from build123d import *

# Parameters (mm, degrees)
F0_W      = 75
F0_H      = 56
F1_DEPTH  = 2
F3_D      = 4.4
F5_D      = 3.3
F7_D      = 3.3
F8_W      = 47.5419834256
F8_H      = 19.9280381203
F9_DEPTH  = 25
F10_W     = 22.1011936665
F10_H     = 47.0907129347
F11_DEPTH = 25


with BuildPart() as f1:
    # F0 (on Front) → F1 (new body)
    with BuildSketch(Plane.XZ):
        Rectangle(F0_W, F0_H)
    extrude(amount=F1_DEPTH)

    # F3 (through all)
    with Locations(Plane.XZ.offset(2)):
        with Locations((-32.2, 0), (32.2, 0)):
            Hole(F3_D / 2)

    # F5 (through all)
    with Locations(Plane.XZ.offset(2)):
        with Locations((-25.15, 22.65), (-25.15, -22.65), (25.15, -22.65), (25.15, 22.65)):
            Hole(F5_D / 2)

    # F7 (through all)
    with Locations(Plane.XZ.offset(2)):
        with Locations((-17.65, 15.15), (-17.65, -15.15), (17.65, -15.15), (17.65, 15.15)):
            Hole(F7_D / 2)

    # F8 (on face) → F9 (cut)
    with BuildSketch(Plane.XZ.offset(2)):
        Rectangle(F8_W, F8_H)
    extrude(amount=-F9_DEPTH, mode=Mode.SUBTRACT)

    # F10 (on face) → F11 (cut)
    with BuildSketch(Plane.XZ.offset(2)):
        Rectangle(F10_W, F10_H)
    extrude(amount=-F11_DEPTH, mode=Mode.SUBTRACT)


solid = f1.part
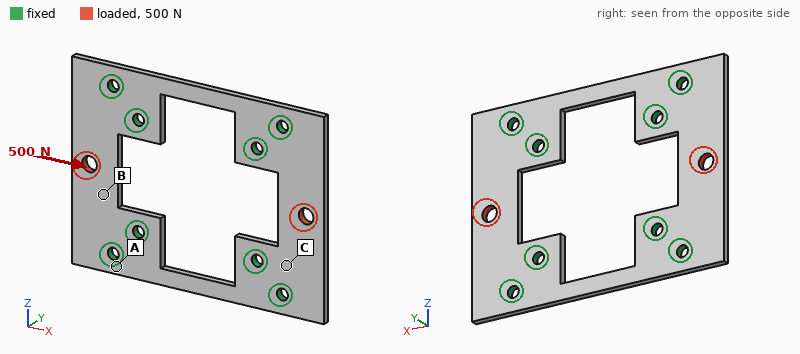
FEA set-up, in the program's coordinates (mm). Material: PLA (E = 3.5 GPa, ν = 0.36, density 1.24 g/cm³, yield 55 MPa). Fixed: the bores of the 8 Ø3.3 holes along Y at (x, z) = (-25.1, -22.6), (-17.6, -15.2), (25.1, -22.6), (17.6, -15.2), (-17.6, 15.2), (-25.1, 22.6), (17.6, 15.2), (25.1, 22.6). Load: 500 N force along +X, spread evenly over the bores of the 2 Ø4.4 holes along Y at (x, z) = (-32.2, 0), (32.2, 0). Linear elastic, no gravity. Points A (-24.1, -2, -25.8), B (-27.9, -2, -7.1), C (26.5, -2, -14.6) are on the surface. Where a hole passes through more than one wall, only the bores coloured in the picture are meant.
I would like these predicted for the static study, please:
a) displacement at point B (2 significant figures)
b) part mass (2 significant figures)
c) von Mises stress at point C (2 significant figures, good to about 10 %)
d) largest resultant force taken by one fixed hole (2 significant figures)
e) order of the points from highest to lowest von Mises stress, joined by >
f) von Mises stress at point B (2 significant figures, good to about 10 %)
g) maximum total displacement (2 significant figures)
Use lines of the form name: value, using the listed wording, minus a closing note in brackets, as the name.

displacement at point B: 54 µm
part mass: 6.3 g
von Mises stress at point C: 4.3 MPa
largest resultant force taken by one fixed hole: 130 N
order of the points from highest to lowest von Mises stress, joined by >: B > C > A
von Mises stress at point B: 11 MPa
maximum total displacement: 97 µm
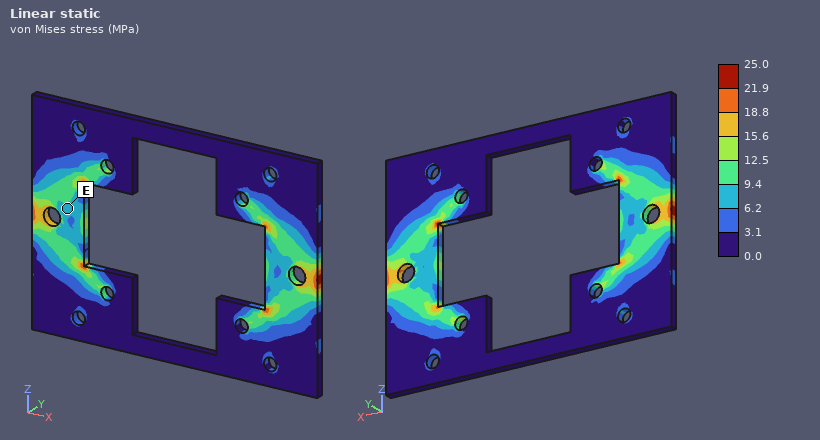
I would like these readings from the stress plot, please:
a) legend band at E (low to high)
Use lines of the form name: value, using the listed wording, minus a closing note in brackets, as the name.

legend band at E: 6.2 to 9.4 MPa
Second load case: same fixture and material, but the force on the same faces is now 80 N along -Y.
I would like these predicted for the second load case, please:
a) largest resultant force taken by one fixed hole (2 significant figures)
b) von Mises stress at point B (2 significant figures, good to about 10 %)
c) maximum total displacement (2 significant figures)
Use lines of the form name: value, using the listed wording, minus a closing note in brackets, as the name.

largest resultant force taken by one fixed hole: 12 N
von Mises stress at point B: 6.1 MPa
maximum total displacement: 0.79 mm
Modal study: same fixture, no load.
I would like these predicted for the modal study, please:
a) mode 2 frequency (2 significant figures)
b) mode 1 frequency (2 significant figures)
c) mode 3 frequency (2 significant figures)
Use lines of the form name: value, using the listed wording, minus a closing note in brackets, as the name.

mode 2 frequency: 1800 Hz
mode 1 frequency: 1800 Hz
mode 3 frequency: 2500 Hz
